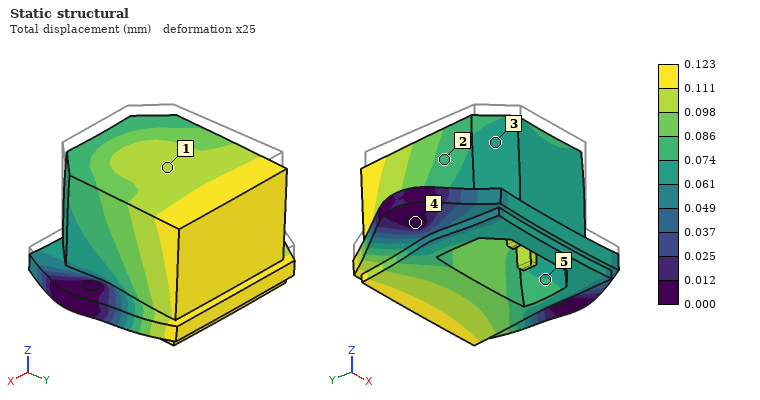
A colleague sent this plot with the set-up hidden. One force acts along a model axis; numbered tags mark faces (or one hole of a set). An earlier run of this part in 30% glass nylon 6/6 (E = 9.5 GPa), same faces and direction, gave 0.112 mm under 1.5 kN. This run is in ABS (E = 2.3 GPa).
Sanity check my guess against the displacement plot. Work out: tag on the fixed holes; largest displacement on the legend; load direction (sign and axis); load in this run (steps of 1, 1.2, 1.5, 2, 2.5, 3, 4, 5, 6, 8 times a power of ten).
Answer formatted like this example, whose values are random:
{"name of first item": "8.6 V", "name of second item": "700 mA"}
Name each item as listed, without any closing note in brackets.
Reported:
{"tag on the fixed holes": "4", "largest displacement on the legend": "0.123 mm", "load direction": "-Z", "load in this run": "400 N"}
